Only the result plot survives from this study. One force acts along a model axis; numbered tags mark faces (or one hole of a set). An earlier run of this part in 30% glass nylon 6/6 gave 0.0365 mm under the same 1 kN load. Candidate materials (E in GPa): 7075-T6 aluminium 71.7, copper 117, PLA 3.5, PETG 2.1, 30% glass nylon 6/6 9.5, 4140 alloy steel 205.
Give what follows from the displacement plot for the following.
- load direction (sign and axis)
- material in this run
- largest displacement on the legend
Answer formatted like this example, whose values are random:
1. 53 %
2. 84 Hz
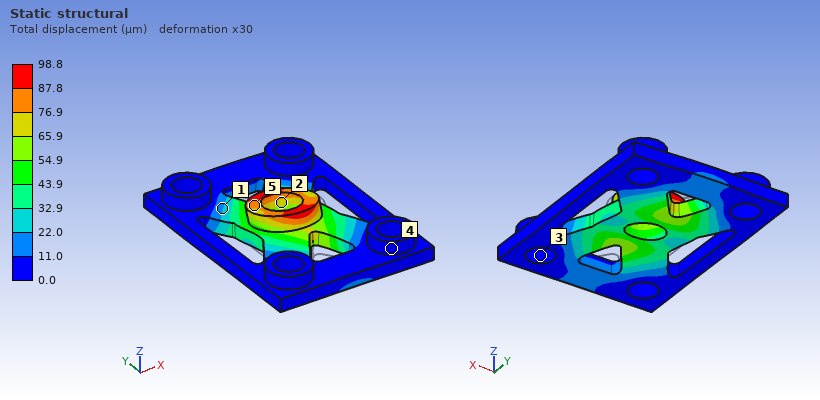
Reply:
1. +Y
2. PLA
3. 98.8 µm
